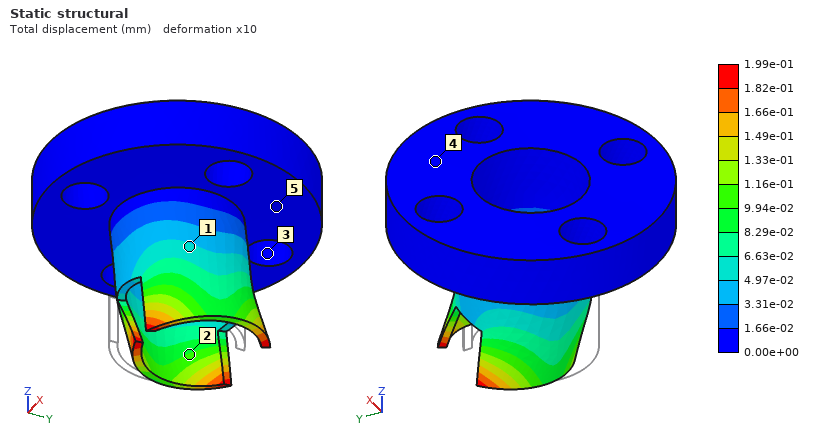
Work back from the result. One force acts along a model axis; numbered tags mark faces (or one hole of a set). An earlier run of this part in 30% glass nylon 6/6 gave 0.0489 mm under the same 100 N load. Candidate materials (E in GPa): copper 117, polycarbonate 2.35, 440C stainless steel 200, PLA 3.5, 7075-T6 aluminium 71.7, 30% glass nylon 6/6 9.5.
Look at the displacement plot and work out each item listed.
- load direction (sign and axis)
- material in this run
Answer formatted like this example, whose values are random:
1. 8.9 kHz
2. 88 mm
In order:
1. +Y
2. polycarbonate
